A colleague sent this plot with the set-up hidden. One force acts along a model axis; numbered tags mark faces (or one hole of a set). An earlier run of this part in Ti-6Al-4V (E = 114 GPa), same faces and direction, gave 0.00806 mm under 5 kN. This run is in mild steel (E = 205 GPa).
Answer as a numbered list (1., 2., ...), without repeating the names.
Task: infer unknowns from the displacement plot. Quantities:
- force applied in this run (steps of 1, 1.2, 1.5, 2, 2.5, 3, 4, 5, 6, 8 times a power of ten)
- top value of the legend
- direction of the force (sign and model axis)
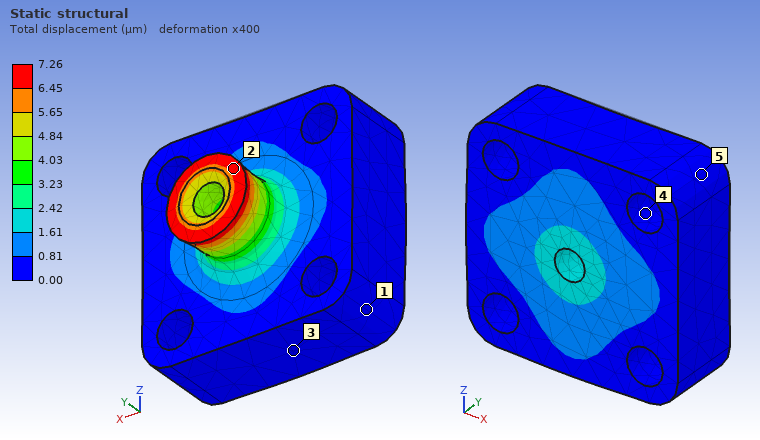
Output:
1. 8 kN
2. 7.26 µm
3. -Y
